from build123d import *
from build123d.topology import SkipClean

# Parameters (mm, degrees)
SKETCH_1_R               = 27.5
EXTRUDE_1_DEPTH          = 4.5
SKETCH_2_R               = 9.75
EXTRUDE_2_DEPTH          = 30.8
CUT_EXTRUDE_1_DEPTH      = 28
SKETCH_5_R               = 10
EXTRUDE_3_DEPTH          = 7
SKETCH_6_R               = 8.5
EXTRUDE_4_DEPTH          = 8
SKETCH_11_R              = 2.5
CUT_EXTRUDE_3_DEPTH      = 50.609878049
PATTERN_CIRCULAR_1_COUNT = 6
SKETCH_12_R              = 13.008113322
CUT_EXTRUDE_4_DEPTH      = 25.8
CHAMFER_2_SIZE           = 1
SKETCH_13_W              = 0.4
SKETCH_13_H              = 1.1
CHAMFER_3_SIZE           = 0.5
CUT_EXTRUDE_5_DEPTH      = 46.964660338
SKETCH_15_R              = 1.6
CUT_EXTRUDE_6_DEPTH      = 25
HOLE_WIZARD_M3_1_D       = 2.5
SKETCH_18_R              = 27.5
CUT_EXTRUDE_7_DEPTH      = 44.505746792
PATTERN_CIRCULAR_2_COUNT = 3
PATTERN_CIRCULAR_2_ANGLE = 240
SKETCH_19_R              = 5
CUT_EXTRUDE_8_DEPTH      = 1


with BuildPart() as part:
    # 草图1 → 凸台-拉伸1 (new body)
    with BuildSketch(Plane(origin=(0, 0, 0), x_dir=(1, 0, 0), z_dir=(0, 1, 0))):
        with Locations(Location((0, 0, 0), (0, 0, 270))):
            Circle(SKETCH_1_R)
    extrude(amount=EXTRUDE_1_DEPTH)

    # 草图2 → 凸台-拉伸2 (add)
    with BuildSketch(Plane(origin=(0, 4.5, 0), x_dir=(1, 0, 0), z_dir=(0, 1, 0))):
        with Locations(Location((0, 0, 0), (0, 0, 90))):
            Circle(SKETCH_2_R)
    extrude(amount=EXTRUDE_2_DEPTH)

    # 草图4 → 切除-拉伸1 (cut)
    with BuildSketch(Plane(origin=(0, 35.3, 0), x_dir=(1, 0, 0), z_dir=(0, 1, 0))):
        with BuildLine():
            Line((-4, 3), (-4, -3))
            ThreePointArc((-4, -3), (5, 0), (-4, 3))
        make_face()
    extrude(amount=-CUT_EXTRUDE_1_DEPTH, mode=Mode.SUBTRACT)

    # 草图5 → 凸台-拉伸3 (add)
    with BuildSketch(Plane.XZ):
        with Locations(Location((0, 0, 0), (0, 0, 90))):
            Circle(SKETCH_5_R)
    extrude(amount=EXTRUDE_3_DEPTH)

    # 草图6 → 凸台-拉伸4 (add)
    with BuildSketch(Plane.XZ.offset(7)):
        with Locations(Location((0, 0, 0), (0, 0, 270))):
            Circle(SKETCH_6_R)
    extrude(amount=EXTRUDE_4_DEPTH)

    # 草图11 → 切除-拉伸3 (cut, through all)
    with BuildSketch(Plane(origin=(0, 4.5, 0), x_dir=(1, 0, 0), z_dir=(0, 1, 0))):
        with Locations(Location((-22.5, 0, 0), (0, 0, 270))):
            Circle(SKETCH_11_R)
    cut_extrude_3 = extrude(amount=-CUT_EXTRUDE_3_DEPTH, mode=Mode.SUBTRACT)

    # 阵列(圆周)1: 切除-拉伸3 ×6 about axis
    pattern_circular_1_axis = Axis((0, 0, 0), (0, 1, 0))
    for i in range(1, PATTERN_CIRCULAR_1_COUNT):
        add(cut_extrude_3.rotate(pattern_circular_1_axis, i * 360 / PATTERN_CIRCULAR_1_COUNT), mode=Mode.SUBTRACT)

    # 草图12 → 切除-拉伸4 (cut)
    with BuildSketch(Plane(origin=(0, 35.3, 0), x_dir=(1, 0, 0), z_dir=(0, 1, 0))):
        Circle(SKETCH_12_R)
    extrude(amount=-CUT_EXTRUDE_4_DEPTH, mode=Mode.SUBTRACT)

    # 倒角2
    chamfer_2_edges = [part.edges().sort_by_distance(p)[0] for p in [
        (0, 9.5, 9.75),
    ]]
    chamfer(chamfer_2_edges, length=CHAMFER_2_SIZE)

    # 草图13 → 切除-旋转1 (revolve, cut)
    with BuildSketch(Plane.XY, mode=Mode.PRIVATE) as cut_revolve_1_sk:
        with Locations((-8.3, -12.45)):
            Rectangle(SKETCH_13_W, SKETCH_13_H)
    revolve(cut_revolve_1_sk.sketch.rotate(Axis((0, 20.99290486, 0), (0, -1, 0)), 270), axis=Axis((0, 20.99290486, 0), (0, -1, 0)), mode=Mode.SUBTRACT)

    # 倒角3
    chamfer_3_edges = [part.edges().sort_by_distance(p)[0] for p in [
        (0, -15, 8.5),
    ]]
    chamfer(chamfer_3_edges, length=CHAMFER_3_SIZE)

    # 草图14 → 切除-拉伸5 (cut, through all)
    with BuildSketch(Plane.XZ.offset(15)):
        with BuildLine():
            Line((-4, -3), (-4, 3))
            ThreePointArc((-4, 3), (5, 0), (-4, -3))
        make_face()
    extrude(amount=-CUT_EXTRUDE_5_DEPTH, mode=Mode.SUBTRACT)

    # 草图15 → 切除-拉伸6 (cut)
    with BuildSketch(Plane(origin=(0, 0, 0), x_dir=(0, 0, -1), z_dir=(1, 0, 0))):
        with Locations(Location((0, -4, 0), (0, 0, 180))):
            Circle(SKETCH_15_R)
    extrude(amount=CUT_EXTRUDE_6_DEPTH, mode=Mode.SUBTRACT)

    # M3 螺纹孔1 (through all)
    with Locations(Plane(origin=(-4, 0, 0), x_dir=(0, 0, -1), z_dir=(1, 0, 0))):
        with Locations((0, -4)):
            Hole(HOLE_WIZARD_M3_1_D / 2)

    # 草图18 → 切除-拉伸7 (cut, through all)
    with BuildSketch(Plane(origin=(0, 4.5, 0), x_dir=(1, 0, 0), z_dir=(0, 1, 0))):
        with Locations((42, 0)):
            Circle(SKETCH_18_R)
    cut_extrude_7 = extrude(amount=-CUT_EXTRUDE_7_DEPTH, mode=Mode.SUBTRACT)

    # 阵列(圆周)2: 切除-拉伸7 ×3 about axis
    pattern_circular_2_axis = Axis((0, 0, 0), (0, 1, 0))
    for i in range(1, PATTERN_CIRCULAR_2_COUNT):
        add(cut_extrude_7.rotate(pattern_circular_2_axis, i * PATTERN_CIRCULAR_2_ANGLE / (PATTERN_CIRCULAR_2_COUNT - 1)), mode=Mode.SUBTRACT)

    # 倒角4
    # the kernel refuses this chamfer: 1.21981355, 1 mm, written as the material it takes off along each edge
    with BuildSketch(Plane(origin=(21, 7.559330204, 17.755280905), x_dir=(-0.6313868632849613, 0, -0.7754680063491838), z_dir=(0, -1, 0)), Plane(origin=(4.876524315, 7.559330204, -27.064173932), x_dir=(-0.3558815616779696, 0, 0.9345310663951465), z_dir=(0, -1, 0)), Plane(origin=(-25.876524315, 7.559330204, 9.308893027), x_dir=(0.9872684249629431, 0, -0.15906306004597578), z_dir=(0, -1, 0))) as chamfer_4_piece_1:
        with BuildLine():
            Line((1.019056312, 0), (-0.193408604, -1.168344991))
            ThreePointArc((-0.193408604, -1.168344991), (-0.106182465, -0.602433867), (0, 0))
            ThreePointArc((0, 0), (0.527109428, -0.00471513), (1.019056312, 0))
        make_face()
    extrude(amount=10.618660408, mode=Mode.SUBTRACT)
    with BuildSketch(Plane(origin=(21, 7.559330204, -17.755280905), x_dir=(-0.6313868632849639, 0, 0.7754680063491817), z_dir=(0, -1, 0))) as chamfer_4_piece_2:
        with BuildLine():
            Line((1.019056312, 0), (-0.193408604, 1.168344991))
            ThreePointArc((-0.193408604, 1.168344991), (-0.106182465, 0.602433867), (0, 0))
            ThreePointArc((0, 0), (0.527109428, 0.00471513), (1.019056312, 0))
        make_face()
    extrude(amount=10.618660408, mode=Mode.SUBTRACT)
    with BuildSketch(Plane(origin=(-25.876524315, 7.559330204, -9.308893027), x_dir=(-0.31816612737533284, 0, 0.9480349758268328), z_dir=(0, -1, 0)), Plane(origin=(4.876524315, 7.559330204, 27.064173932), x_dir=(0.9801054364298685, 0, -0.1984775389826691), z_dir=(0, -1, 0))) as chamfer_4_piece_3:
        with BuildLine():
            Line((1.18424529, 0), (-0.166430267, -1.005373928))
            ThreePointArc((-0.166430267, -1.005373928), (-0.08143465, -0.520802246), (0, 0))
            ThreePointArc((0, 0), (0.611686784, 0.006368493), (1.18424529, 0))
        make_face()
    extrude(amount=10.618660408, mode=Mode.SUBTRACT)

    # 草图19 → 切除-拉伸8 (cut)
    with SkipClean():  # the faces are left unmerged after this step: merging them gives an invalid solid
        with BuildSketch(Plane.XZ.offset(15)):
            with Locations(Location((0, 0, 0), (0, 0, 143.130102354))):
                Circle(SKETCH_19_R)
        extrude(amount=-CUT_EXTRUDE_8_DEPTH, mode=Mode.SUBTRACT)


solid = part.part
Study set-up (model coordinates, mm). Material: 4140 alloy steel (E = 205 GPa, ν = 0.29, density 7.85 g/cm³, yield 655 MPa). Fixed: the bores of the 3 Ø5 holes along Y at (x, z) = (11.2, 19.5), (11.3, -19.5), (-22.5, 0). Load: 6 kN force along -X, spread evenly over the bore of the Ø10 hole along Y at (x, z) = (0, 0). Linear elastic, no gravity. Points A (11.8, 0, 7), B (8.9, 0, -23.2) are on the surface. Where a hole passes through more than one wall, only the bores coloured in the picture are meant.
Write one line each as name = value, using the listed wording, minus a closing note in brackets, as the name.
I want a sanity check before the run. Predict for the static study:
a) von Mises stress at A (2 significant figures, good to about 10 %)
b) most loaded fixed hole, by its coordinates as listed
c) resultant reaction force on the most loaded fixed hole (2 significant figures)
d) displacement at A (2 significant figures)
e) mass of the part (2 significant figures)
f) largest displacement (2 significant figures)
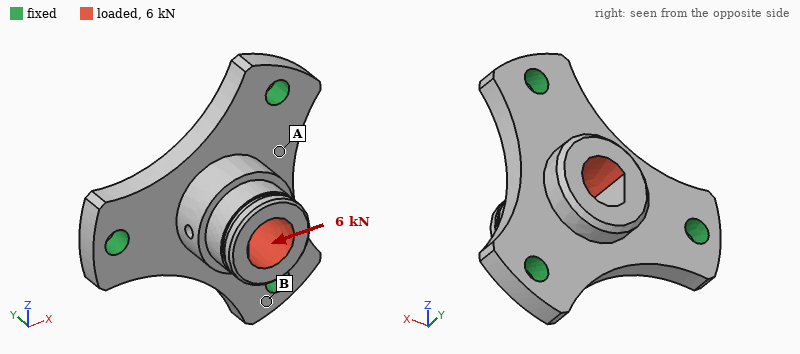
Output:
von Mises stress at A = 59 MPa
most loaded fixed hole, by its coordinates as listed = (-22.5, 0)
resultant reaction force on the most loaded fixed hole = 3.1 kN
displacement at A = 8.2 µm
mass of the part = 76 g
largest displacement = 23 µm
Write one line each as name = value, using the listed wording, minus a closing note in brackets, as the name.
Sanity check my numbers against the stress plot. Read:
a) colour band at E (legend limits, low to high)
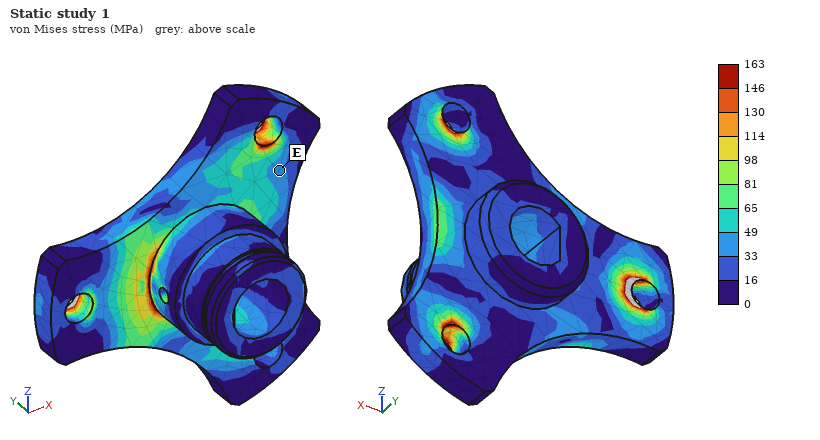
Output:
colour band at E = 33 to 49 MPa
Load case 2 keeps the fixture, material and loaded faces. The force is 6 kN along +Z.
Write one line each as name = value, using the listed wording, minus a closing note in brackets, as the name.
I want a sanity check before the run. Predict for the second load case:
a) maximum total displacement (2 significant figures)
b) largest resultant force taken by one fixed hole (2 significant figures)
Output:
maximum total displacement = 22 µm
largest resultant force taken by one fixed hole = 2.9 kN
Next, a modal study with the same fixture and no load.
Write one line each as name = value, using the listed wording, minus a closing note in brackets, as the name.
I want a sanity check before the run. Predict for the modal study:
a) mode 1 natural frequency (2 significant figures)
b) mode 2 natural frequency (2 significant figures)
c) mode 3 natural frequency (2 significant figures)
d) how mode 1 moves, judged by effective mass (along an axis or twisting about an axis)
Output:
mode 1 natural frequency = 12 kHz
mode 2 natural frequency = 14 kHz
mode 3 natural frequency = 14 kHz
how mode 1 moves, judged by effective mass = along Y
